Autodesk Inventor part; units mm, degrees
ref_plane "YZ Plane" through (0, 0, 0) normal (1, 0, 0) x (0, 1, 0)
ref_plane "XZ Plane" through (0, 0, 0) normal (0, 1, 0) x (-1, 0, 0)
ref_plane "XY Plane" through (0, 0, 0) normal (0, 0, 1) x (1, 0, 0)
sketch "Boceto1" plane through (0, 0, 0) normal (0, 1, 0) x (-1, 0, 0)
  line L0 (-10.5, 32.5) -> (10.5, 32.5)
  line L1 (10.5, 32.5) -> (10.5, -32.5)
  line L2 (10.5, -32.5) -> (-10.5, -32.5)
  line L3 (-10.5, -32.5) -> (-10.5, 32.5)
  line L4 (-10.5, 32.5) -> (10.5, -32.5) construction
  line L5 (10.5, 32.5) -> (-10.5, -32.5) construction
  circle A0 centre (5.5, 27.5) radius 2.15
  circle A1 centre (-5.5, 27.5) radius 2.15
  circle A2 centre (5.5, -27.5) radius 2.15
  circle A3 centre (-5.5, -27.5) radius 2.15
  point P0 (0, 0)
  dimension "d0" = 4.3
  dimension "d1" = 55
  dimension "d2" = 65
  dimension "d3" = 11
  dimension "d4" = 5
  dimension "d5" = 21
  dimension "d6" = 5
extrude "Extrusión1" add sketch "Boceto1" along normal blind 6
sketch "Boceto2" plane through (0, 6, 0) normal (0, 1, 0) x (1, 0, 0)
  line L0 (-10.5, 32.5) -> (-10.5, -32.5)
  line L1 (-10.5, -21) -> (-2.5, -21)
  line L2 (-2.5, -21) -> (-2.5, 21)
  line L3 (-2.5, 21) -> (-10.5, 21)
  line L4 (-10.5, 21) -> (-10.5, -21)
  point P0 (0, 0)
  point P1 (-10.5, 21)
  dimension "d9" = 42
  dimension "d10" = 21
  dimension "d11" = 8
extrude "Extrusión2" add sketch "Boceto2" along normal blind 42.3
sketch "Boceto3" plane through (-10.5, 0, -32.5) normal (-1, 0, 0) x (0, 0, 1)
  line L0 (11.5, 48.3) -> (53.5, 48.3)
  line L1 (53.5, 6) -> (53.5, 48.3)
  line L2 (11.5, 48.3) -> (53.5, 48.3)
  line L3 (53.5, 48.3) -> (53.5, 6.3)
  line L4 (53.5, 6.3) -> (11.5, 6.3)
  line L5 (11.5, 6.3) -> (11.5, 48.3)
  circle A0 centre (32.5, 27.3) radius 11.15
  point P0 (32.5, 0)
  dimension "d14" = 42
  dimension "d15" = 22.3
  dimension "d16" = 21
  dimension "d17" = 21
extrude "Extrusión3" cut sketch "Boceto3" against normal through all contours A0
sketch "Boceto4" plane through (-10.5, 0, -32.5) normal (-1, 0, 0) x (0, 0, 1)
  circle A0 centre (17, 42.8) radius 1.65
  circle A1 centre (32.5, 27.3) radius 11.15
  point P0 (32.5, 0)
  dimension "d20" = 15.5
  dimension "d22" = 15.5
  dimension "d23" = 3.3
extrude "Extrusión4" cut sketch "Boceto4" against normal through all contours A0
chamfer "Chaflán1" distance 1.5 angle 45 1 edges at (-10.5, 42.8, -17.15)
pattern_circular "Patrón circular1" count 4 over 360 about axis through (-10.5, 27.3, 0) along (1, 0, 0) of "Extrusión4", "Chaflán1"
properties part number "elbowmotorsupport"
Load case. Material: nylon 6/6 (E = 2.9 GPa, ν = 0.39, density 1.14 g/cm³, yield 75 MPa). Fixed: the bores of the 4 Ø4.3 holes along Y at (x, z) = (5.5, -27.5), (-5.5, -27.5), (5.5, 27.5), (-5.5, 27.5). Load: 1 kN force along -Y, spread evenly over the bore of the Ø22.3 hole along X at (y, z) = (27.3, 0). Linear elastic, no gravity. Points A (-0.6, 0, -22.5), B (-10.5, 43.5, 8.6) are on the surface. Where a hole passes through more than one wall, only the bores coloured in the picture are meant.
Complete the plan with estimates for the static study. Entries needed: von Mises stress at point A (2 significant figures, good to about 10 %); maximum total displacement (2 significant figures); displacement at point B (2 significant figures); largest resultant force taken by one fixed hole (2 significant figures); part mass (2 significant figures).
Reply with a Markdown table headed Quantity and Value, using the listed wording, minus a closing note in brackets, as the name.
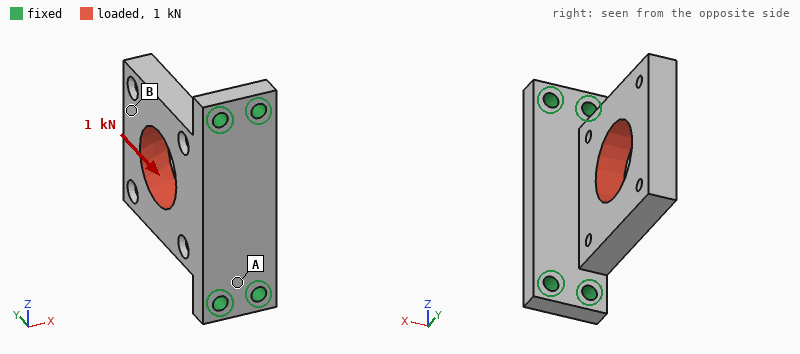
| Quantity | Value |
|---|---|
| von Mises stress at point A | 8.5 MPa |
| maximum total displacement | 0.47 mm |
| displacement at point B | 0.43 mm |
| largest resultant force taken by one fixed hole | 510 N |
| part mass | 21 g |
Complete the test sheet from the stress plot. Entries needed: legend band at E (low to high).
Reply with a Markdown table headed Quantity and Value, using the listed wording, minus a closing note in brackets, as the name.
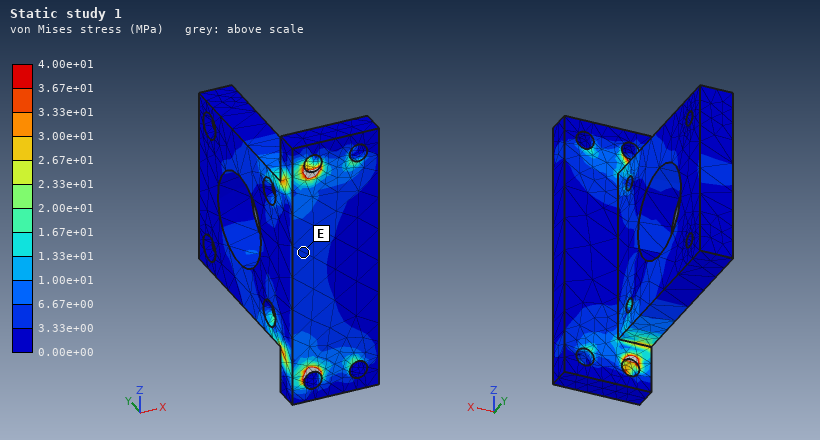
| Quantity | Value |
|---|---|
| legend band at E | 3.33e+00 to 6.67e+00 MPa |
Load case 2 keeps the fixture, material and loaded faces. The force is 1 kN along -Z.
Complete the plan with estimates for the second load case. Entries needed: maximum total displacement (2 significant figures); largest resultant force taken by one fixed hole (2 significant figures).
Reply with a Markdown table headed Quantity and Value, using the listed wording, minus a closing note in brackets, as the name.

| Quantity | Value |
|---|---|
| maximum total displacement | 0.56 mm |
| largest resultant force taken by one fixed hole | 570 N |
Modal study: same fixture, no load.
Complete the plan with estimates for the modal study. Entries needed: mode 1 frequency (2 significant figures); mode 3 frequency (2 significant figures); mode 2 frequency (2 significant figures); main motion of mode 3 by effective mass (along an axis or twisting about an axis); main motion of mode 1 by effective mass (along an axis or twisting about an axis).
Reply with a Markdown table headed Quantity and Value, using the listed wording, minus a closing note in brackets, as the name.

| Quantity | Value |
|---|---|
| mode 1 frequency | 670 Hz |
| mode 3 frequency | 2200 Hz |
| mode 2 frequency | 1800 Hz |
| main motion of mode 3 by effective mass | along Z |
| main motion of mode 1 by effective mass | along X |
